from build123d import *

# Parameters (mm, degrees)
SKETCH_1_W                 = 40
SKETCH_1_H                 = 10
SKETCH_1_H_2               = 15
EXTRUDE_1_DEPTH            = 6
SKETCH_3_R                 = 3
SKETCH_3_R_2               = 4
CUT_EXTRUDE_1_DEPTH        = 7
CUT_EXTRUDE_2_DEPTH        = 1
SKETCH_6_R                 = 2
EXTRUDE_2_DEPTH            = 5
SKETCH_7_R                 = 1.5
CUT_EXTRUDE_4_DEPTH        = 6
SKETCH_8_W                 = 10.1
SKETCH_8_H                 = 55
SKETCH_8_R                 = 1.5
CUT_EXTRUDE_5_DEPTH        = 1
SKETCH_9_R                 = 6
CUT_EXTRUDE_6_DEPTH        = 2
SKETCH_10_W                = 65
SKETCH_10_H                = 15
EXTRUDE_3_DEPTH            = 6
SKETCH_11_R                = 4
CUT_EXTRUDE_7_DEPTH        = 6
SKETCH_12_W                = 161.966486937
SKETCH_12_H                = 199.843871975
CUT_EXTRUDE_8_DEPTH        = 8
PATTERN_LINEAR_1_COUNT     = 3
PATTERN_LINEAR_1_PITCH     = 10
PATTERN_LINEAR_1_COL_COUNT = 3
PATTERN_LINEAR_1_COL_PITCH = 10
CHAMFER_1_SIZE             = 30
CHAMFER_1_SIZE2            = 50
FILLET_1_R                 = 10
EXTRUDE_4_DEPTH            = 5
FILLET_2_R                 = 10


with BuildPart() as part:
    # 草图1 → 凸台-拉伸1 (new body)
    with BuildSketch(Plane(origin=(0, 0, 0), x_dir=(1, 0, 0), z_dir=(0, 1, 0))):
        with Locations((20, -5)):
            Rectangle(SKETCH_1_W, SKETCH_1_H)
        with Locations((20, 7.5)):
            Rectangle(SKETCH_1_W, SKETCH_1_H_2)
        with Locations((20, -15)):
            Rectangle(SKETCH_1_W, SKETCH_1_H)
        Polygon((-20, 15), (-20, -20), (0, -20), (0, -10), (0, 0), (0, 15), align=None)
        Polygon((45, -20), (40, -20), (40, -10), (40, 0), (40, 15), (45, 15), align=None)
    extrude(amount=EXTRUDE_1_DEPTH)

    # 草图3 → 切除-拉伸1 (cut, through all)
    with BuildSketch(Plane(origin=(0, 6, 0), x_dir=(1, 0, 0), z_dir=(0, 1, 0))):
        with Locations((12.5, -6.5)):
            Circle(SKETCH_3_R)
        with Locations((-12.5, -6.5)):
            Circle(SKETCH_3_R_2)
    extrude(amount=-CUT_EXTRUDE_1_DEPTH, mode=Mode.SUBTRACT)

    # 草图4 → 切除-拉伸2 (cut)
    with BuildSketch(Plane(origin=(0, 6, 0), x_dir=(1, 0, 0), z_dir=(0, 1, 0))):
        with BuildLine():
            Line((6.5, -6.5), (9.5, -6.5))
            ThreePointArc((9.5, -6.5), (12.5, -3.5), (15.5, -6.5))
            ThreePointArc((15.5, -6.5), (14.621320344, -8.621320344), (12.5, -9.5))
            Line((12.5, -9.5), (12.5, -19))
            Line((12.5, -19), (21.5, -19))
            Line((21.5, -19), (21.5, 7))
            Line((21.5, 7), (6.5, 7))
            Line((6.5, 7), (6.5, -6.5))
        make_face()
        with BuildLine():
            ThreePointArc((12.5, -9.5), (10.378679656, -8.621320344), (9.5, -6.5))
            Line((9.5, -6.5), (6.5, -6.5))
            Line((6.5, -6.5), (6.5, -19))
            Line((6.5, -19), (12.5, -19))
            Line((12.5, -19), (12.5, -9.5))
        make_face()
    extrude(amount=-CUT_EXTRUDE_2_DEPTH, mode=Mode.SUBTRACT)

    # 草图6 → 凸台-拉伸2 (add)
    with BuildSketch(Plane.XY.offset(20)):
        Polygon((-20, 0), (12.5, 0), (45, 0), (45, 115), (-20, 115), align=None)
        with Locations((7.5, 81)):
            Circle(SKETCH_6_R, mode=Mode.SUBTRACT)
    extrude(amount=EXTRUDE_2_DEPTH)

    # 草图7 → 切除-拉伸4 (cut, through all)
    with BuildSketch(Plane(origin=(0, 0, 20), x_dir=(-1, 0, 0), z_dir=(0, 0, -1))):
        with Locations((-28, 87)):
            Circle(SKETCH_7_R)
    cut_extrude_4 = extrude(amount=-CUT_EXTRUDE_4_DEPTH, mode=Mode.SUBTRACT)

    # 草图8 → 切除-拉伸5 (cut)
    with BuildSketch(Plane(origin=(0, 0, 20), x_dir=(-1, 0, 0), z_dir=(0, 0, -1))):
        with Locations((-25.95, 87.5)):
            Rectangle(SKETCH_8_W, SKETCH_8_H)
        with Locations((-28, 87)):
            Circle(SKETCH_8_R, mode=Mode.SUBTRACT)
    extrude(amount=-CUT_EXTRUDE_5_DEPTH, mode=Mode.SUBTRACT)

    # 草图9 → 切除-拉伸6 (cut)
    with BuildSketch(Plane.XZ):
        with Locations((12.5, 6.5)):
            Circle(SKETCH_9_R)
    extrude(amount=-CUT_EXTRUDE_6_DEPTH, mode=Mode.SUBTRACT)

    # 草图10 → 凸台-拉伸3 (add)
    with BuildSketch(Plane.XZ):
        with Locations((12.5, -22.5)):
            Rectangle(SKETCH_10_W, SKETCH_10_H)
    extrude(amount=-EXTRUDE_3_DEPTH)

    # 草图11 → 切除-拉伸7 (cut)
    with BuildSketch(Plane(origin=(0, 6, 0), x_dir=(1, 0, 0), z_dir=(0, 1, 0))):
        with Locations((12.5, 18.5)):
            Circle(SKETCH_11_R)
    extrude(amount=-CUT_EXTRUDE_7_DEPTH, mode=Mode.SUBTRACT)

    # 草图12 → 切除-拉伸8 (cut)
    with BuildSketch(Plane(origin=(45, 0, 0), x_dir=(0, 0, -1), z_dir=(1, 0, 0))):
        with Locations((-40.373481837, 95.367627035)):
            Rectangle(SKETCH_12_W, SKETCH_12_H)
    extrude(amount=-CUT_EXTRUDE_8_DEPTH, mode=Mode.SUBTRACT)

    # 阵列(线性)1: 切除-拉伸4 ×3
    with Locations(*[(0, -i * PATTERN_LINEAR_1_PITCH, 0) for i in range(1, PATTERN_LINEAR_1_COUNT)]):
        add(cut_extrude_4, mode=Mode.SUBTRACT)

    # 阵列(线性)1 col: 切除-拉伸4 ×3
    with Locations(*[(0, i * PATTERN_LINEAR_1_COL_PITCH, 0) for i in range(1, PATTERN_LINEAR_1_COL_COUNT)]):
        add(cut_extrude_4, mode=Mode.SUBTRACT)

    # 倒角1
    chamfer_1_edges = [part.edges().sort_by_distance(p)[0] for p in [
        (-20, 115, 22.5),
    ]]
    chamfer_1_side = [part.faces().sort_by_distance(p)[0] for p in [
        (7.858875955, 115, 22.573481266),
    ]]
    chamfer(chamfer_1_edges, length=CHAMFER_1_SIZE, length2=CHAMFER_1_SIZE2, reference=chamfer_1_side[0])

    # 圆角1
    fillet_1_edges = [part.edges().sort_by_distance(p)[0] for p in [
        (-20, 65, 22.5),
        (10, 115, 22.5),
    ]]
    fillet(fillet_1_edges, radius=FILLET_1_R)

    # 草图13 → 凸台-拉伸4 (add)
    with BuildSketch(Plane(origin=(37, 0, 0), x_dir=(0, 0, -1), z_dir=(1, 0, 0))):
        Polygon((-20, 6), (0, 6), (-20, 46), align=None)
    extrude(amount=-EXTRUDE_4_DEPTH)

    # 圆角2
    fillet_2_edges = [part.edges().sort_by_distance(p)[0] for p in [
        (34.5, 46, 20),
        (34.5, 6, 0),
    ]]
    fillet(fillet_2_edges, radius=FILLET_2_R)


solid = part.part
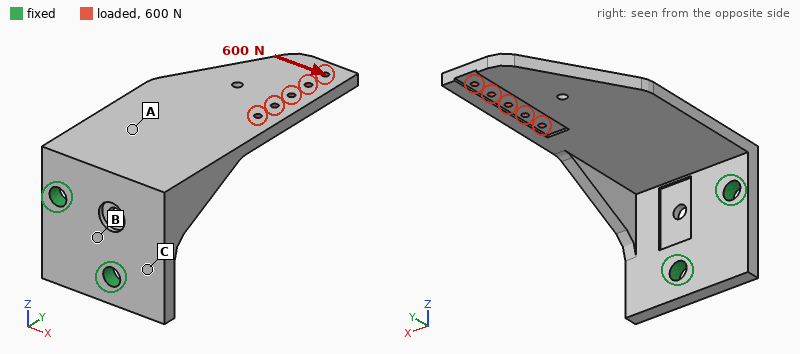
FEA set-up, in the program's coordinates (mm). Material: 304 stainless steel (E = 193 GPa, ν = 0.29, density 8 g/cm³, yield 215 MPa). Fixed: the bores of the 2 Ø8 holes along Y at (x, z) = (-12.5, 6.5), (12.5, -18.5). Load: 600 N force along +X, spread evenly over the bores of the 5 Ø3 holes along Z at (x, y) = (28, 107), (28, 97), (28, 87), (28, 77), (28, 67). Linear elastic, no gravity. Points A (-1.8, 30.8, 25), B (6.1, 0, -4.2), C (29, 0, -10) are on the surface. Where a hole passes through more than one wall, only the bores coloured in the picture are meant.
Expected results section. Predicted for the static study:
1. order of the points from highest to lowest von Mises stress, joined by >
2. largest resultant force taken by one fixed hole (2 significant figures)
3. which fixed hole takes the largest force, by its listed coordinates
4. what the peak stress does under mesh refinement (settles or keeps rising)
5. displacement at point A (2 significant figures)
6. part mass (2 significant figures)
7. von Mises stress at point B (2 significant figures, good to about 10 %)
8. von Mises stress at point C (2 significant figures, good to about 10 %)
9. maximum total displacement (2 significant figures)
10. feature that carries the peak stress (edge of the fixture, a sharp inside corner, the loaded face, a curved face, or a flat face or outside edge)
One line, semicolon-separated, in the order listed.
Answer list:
C > B > A; 880 N; (-12.5, 6.5); keeps rising; 0.090 mm; 370 g; 48 MPa; 67 MPa; 0.45 mm; edge of the fixture
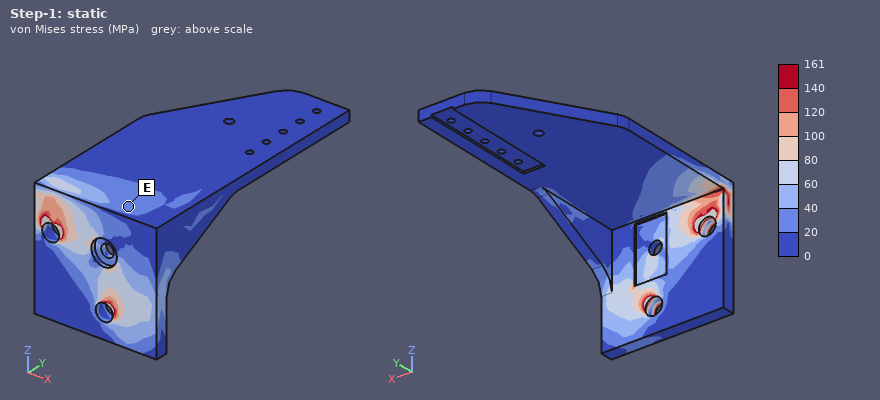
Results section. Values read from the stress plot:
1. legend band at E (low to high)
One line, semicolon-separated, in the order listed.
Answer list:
20 to 40 MPa
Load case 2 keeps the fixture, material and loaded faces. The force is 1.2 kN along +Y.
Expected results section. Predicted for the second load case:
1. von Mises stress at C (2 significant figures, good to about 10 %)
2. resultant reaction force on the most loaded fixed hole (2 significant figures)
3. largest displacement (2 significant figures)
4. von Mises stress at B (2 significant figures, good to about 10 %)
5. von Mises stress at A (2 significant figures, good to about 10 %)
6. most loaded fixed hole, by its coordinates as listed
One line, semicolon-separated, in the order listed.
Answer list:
70 MPa; 760 N; 0.49 mm; 53 MPa; 13 MPa; (-12.5, 6.5)
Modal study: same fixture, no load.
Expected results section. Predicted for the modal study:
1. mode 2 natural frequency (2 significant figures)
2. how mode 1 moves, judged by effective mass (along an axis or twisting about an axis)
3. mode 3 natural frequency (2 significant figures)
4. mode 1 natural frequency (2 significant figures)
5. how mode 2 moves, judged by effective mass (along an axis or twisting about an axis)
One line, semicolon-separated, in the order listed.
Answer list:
840 Hz; along Z; 1600 Hz; 400 Hz; along X
